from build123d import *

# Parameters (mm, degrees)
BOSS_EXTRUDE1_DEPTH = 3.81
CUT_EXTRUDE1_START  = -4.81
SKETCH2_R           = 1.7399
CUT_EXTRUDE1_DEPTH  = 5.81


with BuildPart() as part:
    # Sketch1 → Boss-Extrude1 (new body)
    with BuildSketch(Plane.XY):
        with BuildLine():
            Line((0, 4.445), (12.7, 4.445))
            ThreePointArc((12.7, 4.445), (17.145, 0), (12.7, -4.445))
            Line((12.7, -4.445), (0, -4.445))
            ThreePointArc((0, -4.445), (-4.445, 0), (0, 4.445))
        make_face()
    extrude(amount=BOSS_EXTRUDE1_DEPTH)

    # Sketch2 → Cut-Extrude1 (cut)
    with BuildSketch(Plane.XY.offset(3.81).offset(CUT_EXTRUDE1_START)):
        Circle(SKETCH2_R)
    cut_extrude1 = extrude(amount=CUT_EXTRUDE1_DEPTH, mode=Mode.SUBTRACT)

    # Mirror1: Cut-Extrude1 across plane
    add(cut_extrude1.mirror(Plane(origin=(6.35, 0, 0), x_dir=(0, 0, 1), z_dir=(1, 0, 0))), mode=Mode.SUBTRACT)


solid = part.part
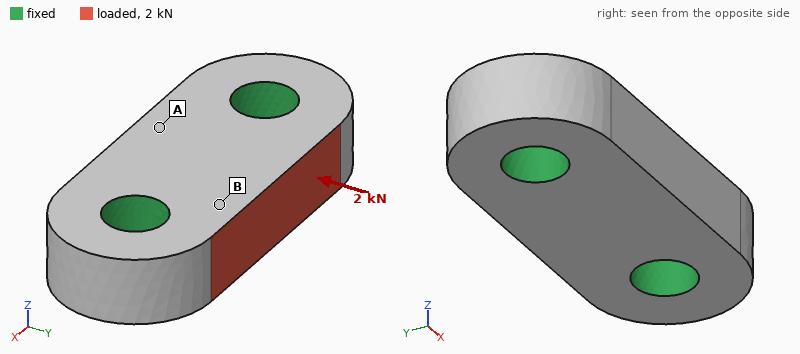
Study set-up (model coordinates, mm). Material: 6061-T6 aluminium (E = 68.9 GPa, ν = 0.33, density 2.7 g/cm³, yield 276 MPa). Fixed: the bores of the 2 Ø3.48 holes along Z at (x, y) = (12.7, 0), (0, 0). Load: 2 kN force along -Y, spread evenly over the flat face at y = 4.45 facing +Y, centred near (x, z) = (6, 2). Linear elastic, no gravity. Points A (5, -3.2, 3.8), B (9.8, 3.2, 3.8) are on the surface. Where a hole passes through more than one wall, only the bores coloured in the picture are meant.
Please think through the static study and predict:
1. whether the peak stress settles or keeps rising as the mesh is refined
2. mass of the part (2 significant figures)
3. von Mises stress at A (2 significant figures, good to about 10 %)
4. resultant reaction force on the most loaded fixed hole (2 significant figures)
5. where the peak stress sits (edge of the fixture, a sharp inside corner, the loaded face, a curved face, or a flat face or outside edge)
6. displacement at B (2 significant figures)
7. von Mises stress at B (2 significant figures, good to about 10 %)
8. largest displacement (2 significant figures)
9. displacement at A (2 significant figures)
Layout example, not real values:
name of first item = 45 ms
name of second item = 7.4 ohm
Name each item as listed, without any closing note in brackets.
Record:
whether the peak stress settles or keeps rising as the mesh is refined = keeps rising
mass of the part = 1.6 g
von Mises stress at A = 19 MPa
resultant reaction force on the most loaded fixed hole = 1.0 kN
where the peak stress sits = edge of the fixture
displacement at B = 3.3 µm
von Mises stress at B = 42 MPa
largest displacement = 5.4 µm
displacement at A = 2.9 µm
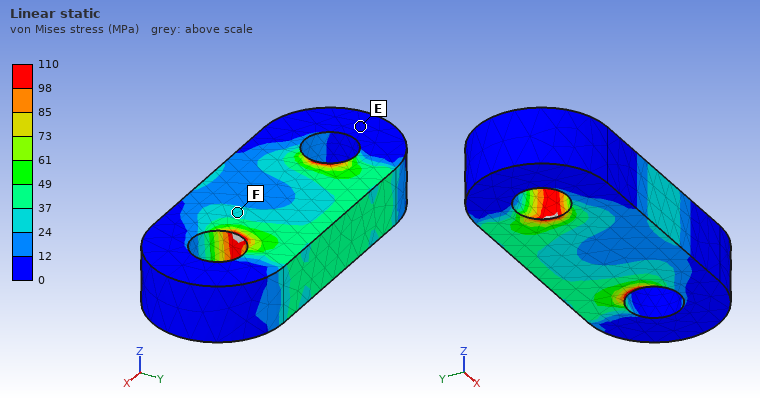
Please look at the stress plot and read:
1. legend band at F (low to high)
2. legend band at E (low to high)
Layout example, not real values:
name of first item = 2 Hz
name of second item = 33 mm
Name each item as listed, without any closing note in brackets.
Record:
legend band at F = 24 to 37 MPa
legend band at E = 0 to 12 MPa
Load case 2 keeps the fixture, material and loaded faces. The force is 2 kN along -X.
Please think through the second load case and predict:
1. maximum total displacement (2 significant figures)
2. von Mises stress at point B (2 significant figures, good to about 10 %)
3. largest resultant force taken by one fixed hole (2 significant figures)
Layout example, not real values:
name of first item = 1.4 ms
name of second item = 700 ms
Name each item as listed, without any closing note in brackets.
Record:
maximum total displacement = 5.4 µm
von Mises stress at point B = 66 MPa
largest resultant force taken by one fixed hole = 1.1 kN
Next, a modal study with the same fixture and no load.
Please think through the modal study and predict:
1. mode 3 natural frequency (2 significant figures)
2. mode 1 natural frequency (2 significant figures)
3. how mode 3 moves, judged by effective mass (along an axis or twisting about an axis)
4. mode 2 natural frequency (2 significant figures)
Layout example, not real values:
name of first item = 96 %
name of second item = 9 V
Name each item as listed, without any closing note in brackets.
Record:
mode 3 natural frequency = 120 kHz
mode 1 natural frequency = 98 kHz
how mode 3 moves, judged by effective mass = along Y
mode 2 natural frequency = 99 kHz
